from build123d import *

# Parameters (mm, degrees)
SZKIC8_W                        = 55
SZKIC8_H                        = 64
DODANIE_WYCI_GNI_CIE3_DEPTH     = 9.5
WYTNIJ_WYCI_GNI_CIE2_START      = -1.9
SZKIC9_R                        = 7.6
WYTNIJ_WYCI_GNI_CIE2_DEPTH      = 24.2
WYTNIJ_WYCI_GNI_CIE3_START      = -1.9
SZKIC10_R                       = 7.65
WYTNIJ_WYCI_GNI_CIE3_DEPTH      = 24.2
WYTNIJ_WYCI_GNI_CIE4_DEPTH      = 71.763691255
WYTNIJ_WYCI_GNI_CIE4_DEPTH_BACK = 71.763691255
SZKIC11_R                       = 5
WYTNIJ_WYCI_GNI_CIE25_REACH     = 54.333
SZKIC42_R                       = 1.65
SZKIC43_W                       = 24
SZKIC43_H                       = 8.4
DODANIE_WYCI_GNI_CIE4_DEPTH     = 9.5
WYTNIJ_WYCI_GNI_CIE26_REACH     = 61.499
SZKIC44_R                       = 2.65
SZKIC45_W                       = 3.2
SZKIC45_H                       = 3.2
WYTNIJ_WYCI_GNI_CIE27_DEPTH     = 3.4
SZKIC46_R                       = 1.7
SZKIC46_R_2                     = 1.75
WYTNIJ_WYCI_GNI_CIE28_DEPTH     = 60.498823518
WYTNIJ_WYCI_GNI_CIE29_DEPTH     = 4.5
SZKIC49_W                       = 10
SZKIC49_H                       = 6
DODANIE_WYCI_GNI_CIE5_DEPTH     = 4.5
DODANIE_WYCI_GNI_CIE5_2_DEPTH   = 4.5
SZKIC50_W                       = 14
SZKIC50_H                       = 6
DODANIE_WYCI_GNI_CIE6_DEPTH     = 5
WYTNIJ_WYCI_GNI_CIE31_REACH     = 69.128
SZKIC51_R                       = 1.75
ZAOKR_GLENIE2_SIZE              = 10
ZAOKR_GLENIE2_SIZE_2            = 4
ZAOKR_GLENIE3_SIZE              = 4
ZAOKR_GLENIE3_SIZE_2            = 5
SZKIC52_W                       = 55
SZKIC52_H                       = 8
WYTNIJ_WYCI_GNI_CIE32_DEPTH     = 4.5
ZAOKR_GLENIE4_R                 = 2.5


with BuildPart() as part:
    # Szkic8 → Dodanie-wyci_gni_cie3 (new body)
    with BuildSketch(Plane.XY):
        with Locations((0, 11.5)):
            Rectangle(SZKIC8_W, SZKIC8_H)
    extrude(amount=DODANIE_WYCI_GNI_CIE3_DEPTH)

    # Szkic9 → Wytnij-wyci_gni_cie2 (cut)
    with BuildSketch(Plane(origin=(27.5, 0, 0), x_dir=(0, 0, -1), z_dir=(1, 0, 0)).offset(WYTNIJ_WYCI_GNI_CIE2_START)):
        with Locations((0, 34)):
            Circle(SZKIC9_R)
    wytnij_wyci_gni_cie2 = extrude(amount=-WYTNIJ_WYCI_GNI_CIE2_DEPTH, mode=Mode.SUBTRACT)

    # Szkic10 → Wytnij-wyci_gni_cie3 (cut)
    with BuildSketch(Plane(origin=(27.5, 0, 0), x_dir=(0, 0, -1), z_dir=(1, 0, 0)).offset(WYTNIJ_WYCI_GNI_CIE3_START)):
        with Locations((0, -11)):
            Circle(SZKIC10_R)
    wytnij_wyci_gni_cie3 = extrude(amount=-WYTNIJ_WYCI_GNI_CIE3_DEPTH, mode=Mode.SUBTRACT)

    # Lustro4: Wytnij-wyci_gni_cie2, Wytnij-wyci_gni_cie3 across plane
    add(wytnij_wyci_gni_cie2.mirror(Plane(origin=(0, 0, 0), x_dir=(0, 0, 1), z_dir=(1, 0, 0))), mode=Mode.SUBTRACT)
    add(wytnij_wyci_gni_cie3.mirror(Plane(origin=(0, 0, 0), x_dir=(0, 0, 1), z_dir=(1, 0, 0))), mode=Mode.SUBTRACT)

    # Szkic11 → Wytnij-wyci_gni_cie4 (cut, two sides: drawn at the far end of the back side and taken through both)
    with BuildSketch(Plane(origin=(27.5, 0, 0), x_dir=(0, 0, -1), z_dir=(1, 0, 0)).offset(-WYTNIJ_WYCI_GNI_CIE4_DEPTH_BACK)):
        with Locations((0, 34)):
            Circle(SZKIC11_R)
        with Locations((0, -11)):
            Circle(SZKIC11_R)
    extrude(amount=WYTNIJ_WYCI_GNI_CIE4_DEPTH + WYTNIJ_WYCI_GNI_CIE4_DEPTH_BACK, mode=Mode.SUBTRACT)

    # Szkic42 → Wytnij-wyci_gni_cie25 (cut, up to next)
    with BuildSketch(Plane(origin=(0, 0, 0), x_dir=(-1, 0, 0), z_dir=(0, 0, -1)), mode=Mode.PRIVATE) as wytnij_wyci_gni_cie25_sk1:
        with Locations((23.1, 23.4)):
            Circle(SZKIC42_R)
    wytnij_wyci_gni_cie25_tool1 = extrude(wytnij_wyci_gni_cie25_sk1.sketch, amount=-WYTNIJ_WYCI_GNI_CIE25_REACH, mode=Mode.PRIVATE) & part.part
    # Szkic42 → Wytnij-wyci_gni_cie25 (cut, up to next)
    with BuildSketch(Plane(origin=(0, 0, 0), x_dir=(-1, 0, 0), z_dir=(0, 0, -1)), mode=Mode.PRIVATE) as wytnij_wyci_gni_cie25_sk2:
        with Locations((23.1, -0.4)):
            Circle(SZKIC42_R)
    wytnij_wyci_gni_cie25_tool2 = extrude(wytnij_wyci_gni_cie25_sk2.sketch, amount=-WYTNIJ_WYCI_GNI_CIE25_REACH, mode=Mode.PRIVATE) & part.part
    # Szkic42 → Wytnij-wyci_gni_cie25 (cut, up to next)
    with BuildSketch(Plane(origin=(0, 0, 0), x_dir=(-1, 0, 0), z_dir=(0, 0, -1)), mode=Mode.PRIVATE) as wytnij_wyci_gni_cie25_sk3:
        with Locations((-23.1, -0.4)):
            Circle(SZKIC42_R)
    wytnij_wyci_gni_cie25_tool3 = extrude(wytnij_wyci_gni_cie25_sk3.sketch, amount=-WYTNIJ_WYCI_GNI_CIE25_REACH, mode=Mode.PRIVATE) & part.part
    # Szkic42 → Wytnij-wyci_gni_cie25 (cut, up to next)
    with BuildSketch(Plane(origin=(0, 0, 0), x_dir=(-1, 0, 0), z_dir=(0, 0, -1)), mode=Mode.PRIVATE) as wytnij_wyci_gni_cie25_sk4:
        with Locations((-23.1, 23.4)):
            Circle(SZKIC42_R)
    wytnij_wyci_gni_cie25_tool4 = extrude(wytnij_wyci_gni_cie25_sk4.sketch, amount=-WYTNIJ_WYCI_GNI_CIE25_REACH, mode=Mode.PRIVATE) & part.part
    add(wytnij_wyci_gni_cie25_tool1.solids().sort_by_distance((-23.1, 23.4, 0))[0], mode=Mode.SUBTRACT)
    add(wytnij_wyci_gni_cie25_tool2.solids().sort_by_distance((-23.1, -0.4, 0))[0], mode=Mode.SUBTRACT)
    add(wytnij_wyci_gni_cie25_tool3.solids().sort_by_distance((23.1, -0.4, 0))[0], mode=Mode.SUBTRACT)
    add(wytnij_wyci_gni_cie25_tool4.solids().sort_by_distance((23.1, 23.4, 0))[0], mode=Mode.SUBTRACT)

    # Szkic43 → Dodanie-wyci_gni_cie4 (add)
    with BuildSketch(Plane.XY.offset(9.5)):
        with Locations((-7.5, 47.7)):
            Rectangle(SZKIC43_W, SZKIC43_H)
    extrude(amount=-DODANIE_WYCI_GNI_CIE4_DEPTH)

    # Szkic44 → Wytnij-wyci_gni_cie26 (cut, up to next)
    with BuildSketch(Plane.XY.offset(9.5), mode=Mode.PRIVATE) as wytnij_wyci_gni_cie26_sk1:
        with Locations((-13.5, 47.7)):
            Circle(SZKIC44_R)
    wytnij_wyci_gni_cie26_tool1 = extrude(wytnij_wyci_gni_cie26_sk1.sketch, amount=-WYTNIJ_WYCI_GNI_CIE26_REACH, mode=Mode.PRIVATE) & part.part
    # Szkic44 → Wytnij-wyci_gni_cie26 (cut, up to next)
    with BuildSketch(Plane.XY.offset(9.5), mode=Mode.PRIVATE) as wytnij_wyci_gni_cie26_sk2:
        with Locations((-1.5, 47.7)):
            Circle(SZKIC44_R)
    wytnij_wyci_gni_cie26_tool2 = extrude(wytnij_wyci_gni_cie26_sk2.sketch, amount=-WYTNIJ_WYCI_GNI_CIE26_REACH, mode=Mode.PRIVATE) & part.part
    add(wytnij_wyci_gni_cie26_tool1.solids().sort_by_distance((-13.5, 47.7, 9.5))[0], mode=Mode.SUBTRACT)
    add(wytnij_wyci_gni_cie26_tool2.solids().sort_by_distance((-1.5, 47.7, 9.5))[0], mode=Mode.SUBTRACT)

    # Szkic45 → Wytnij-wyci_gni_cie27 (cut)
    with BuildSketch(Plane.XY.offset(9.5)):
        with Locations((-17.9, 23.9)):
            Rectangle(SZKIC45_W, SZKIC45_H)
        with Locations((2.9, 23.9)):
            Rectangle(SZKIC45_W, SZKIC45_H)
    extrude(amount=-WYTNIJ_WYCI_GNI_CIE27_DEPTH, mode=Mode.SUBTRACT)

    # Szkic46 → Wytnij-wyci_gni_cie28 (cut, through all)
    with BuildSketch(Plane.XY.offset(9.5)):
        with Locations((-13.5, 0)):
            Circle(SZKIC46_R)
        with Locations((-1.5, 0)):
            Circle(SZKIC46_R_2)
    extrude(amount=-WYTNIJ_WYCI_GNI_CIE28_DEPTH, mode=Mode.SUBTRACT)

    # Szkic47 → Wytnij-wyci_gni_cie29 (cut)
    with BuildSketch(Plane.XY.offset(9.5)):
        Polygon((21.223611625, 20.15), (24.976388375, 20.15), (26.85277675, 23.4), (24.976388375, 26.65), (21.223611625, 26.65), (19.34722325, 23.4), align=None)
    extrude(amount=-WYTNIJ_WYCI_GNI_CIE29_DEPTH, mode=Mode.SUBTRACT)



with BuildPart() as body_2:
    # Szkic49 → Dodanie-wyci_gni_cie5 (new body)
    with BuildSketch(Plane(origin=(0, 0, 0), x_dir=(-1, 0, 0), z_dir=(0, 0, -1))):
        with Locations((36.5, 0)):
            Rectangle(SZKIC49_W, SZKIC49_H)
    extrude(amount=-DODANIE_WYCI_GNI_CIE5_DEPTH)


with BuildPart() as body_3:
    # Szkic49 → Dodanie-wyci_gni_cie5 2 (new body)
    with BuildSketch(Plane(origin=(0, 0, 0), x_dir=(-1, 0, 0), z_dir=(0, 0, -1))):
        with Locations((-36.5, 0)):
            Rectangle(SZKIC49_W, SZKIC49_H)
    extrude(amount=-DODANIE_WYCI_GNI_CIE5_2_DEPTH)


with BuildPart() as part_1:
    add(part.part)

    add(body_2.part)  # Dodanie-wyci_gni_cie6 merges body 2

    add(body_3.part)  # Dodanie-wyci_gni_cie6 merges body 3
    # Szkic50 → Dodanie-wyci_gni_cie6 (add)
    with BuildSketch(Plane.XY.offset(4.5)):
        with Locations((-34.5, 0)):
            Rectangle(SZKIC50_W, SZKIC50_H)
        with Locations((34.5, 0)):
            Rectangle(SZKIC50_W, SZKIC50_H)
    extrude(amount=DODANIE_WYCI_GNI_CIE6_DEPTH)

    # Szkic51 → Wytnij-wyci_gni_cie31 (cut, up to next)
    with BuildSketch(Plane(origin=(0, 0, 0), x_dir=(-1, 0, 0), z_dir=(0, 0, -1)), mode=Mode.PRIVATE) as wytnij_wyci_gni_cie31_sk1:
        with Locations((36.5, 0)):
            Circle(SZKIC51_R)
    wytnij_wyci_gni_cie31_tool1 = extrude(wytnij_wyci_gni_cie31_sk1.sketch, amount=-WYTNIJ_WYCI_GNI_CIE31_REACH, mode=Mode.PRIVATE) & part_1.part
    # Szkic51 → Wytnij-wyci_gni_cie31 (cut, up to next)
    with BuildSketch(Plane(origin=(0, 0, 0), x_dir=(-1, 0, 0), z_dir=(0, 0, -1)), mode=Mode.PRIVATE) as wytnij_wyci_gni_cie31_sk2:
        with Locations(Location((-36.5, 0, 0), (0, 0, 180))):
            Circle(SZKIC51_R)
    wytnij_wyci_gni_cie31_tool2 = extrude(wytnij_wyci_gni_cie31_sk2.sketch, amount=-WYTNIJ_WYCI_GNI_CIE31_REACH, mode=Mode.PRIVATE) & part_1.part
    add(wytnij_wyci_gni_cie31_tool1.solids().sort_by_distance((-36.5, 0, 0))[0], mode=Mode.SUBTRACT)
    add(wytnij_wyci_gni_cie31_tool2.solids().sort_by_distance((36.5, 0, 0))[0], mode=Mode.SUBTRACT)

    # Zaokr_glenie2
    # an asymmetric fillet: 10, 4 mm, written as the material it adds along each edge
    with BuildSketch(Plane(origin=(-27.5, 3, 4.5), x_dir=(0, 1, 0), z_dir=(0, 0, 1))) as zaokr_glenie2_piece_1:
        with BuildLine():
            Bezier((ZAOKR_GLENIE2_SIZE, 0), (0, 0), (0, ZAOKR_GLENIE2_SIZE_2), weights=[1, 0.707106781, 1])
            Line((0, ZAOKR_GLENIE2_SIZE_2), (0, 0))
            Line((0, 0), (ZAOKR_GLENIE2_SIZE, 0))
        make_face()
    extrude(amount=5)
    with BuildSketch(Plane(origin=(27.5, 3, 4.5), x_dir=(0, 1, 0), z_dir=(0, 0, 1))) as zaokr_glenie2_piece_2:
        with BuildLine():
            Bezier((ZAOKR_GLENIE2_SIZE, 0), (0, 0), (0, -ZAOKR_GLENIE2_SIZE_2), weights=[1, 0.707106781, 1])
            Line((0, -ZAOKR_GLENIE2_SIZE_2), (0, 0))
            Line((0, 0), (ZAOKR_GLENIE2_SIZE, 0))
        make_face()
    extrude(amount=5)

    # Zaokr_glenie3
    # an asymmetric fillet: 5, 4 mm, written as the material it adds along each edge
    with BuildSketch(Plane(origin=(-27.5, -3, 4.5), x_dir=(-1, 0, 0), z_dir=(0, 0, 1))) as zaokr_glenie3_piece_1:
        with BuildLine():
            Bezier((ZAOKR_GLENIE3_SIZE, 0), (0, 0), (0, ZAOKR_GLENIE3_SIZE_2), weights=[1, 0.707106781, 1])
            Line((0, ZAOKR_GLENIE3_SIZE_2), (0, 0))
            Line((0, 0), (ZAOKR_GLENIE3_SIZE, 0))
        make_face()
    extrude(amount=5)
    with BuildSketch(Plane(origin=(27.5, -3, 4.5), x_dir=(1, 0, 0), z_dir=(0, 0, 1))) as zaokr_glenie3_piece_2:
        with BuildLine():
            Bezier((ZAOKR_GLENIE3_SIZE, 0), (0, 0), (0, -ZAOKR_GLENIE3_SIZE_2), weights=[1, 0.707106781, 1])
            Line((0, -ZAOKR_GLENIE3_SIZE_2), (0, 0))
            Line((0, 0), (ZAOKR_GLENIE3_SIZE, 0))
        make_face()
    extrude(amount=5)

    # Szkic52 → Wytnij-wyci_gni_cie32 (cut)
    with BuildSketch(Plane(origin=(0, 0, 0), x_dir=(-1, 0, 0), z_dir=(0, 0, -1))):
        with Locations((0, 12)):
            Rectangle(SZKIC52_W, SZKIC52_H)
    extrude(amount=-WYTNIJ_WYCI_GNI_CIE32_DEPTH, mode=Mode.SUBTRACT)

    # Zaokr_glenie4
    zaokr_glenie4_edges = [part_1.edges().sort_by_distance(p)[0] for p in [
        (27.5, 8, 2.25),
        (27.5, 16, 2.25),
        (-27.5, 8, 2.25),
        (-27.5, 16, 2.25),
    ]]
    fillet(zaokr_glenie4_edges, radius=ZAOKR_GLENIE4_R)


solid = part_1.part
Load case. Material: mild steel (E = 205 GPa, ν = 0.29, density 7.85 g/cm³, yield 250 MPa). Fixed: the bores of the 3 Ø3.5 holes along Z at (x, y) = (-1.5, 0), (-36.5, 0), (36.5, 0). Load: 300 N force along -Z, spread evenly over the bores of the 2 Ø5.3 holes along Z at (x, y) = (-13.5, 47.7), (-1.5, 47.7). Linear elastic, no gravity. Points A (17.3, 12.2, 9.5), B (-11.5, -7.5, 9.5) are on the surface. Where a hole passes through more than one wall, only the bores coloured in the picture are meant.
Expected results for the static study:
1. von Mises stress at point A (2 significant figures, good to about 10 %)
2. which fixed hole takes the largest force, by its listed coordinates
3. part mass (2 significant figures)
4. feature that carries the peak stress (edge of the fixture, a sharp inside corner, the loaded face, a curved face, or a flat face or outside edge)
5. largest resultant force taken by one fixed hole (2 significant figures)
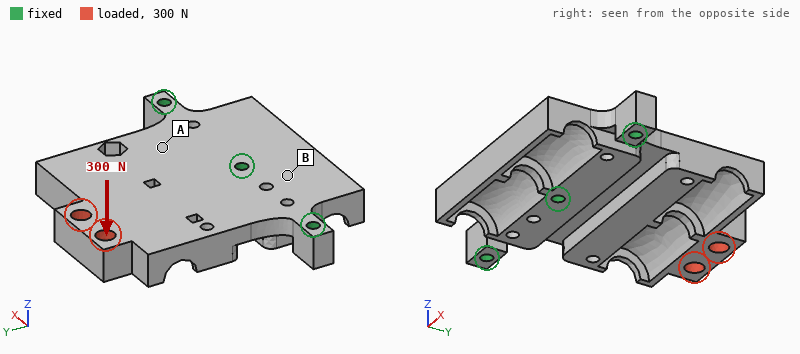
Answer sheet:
37 MPa
(-1.5, 0)
190 g
a curved face
350 N
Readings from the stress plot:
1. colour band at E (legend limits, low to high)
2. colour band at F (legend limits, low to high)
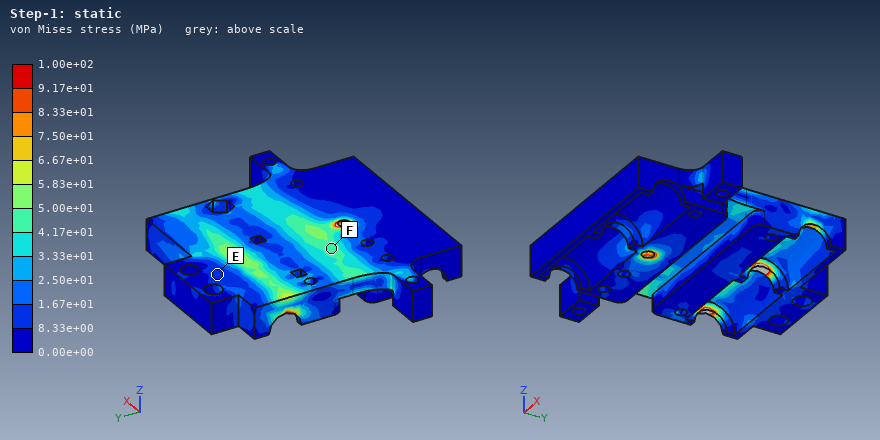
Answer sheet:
8.33e+00 to 1.67e+01 MPa
4.17e+01 to 5.00e+01 MPa
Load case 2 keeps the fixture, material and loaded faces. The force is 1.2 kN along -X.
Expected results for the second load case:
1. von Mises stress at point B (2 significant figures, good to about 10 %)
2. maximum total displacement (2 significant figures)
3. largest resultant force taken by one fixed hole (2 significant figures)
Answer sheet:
7.1 MPa
21 µm
900 N
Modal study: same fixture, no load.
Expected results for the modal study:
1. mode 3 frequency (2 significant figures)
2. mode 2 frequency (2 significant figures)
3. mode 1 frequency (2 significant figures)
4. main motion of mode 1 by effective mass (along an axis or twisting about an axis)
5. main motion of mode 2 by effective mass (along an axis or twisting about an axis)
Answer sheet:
6000 Hz
4500 Hz
1800 Hz
along Z
twisting about Y
